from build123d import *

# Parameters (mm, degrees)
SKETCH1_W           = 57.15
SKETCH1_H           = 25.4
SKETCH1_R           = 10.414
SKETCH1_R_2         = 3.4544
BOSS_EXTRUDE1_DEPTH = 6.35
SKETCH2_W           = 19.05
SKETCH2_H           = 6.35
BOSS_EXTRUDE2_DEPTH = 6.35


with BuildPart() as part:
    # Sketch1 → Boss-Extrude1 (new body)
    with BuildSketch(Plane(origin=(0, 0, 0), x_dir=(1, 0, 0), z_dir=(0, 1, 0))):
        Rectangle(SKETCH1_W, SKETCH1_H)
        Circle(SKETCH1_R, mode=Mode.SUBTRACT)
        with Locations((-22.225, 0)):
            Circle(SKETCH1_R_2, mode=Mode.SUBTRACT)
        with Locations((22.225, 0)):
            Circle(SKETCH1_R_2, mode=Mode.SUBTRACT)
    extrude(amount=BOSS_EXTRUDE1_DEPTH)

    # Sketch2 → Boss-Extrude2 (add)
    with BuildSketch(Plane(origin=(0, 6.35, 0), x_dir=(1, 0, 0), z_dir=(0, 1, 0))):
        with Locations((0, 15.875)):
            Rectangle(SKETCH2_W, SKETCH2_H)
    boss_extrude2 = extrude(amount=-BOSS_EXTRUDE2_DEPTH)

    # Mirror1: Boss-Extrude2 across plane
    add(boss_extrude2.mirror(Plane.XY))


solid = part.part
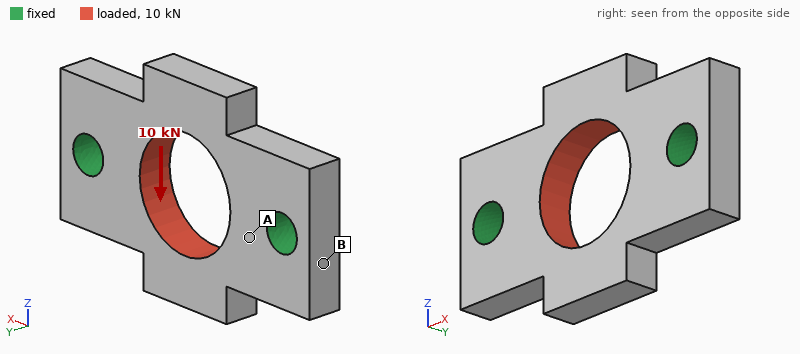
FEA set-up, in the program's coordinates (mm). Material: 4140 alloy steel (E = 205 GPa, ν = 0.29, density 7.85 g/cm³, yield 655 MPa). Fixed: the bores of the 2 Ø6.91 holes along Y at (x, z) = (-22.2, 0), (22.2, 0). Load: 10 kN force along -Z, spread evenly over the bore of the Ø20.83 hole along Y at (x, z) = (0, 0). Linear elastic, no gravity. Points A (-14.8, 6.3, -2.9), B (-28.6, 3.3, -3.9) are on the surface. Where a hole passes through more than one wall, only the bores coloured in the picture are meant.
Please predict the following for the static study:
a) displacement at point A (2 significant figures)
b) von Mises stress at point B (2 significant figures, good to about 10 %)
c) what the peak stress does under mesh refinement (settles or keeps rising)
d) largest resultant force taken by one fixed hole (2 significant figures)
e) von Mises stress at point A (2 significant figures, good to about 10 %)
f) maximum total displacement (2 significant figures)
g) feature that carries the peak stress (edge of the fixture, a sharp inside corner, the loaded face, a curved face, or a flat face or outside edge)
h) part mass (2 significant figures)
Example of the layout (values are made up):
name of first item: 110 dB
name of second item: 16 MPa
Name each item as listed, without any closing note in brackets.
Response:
displacement at point A: 4.1 µm
von Mises stress at point B: 25 MPa
what the peak stress does under mesh refinement: keeps rising
largest resultant force taken by one fixed hole: 5.0 kN
von Mises stress at point A: 73 MPa
maximum total displacement: 9.7 µm
feature that carries the peak stress: edge of the fixture
part mass: 64 g
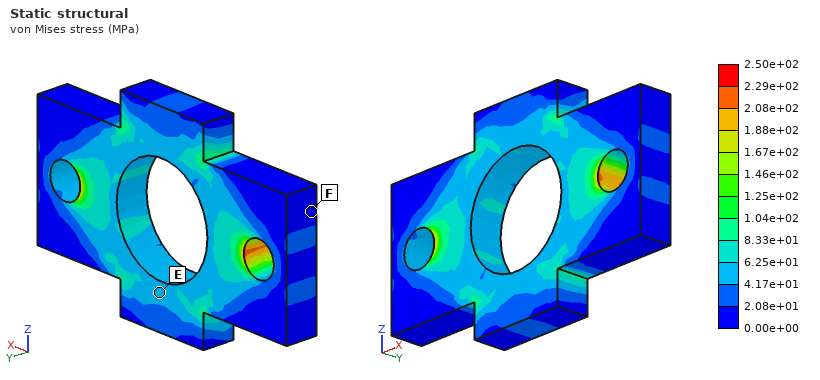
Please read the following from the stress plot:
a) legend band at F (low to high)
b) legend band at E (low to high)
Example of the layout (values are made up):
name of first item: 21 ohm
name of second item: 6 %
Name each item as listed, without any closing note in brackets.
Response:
legend band at F: 0.00e+00 to 2.08e+01 MPa
legend band at E: 4.17e+01 to 6.25e+01 MPa
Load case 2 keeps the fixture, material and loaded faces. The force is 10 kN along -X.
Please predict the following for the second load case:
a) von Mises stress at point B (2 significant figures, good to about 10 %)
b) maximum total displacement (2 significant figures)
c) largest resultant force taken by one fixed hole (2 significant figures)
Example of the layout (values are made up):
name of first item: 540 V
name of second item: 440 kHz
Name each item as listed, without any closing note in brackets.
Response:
von Mises stress at point B: 28 MPa
maximum total displacement: 5.1 µm
largest resultant force taken by one fixed hole: 5.0 kN
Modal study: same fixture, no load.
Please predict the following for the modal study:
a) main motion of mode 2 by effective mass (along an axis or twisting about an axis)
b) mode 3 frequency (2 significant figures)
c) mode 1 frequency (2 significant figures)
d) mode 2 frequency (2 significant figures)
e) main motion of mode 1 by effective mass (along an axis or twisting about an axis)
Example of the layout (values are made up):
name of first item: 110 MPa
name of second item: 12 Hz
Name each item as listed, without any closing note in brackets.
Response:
main motion of mode 2 by effective mass: along Y
mode 3 frequency: 27 kHz
mode 1 frequency: 11 kHz
mode 2 frequency: 12 kHz
main motion of mode 1 by effective mass: twisting about X
